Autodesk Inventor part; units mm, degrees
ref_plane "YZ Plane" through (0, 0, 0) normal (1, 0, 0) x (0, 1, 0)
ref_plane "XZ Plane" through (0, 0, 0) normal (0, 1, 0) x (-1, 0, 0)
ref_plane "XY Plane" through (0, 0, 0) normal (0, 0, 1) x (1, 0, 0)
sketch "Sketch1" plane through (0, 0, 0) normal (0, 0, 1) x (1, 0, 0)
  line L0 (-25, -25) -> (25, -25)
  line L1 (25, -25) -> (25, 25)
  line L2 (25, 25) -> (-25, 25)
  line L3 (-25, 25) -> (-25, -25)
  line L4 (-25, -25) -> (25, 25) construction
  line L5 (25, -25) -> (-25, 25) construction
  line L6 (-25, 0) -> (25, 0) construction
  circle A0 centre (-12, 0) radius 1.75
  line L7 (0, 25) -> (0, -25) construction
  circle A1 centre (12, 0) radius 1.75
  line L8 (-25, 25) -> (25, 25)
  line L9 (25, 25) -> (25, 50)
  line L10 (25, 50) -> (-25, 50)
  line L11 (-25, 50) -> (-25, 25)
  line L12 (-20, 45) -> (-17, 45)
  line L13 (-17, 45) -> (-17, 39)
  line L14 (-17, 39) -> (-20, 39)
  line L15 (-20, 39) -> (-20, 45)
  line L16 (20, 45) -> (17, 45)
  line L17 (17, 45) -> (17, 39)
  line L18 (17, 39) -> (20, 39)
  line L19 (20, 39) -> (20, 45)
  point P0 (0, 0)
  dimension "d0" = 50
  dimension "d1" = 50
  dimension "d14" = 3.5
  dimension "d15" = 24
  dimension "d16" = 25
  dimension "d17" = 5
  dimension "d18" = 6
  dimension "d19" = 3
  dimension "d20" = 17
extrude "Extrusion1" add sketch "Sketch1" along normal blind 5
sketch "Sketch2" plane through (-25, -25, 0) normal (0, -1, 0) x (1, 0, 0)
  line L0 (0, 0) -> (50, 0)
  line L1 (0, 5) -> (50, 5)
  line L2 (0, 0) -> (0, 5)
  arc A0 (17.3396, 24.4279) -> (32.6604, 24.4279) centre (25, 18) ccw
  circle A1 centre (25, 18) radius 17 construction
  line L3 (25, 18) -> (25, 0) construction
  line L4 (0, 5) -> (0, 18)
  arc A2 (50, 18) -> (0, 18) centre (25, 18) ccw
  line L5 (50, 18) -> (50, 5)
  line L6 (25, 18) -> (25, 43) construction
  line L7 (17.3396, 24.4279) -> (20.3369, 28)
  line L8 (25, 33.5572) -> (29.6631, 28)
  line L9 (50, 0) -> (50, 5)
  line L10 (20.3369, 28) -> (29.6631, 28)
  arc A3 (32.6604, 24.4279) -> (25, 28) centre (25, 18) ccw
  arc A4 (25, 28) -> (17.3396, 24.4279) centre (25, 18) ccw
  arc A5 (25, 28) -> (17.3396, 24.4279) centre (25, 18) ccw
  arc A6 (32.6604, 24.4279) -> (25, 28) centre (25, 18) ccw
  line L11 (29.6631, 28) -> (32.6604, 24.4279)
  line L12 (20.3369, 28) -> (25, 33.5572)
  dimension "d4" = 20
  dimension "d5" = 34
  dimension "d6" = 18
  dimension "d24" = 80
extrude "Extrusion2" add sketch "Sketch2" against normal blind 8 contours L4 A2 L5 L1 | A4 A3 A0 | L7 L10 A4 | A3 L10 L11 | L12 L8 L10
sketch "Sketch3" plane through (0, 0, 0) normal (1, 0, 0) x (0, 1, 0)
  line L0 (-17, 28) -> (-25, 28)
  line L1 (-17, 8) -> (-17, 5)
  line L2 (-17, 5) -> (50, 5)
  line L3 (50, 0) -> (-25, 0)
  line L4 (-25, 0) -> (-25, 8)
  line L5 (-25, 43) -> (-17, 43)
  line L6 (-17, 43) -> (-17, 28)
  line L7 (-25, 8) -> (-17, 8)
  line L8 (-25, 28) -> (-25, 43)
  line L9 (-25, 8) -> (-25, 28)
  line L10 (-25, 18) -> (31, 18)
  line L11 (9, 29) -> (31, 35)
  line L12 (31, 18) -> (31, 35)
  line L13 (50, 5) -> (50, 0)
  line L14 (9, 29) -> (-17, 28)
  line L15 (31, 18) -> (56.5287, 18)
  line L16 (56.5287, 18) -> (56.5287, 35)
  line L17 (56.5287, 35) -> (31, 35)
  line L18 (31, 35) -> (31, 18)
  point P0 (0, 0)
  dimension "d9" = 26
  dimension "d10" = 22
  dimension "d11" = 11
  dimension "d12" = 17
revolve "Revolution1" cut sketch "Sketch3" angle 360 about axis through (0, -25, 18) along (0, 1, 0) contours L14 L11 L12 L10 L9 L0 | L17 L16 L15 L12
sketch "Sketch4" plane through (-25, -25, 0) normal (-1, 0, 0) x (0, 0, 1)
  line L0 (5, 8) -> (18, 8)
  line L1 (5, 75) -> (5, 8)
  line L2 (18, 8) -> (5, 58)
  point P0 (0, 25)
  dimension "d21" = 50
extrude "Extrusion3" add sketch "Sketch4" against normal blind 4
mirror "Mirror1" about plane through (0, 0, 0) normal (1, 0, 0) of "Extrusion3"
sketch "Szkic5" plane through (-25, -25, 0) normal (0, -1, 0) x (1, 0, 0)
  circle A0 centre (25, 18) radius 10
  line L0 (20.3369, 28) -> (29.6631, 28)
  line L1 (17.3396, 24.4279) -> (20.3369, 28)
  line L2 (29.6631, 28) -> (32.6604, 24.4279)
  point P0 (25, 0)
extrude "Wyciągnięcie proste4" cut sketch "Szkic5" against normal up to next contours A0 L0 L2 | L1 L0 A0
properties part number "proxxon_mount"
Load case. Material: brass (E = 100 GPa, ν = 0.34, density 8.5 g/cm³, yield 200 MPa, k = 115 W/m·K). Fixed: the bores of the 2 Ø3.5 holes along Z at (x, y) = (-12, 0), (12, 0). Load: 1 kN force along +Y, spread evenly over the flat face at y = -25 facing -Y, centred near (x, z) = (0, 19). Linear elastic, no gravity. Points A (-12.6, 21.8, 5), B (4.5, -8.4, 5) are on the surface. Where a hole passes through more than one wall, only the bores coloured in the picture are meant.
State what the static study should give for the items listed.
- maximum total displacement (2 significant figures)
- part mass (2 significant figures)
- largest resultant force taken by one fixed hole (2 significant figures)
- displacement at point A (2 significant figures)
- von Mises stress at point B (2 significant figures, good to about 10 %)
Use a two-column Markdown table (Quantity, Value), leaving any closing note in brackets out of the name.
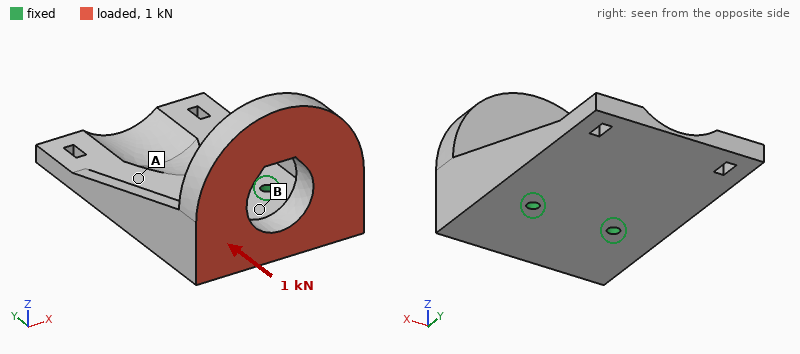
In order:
| Quantity | Value |
|---|---|
| maximum total displacement | 0.13 mm |
| part mass | 260 g |
| largest resultant force taken by one fixed hole | 510 N |
| displacement at point A | 0.030 mm |
| von Mises stress at point B | 27 MPa |
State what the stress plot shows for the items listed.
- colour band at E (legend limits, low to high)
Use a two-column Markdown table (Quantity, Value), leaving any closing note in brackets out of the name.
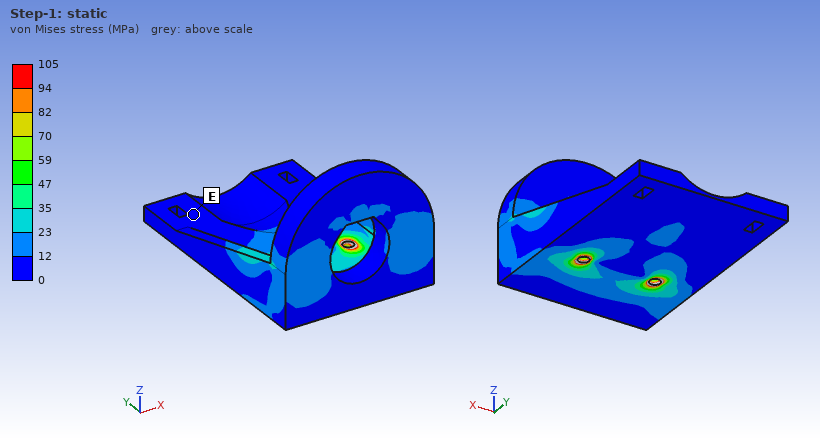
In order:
| Quantity | Value |
|---|---|
| colour band at E | 0 to 12 MPa |
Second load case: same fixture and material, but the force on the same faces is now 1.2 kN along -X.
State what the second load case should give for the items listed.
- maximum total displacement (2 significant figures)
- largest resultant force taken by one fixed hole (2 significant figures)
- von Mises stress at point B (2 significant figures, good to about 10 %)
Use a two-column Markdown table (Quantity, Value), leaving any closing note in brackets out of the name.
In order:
| Quantity | Value |
|---|---|
| maximum total displacement | 56 µm |
| largest resultant force taken by one fixed hole | 1.4 kN |
| von Mises stress at point B | 33 MPa |
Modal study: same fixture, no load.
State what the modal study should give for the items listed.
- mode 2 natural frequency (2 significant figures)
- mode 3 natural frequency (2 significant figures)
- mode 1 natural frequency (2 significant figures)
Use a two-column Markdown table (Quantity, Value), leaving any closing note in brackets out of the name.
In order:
| Quantity | Value |
|---|---|
| mode 2 natural frequency | 2100 Hz |
| mode 3 natural frequency | 2200 Hz |
| mode 1 natural frequency | 1200 Hz |
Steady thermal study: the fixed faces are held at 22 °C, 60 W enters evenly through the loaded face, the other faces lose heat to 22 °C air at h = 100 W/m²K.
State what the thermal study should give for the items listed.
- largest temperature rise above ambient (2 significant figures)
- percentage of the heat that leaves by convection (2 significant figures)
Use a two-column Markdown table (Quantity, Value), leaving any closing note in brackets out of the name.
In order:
| Quantity | Value |
|---|---|
| largest temperature rise above ambient | 51 K |
| percentage of the heat that leaves by convection | 33 % |
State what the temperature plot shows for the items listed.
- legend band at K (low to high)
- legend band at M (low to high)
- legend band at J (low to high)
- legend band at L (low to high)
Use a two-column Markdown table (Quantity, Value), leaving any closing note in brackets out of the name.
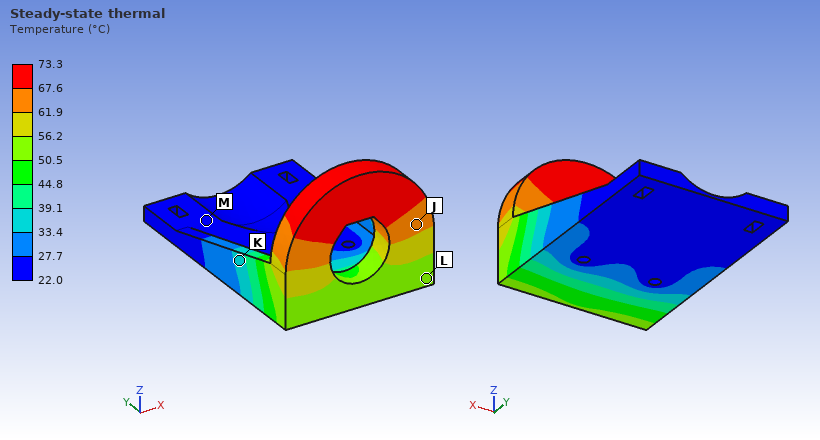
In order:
| Quantity | Value |
|---|---|
| legend band at K | 33.4 to 39.1 °C |
| legend band at M | 22.0 to 27.7 °C |
| legend band at J | 61.9 to 67.6 °C |
| legend band at L | 50.5 to 56.2 °C |
